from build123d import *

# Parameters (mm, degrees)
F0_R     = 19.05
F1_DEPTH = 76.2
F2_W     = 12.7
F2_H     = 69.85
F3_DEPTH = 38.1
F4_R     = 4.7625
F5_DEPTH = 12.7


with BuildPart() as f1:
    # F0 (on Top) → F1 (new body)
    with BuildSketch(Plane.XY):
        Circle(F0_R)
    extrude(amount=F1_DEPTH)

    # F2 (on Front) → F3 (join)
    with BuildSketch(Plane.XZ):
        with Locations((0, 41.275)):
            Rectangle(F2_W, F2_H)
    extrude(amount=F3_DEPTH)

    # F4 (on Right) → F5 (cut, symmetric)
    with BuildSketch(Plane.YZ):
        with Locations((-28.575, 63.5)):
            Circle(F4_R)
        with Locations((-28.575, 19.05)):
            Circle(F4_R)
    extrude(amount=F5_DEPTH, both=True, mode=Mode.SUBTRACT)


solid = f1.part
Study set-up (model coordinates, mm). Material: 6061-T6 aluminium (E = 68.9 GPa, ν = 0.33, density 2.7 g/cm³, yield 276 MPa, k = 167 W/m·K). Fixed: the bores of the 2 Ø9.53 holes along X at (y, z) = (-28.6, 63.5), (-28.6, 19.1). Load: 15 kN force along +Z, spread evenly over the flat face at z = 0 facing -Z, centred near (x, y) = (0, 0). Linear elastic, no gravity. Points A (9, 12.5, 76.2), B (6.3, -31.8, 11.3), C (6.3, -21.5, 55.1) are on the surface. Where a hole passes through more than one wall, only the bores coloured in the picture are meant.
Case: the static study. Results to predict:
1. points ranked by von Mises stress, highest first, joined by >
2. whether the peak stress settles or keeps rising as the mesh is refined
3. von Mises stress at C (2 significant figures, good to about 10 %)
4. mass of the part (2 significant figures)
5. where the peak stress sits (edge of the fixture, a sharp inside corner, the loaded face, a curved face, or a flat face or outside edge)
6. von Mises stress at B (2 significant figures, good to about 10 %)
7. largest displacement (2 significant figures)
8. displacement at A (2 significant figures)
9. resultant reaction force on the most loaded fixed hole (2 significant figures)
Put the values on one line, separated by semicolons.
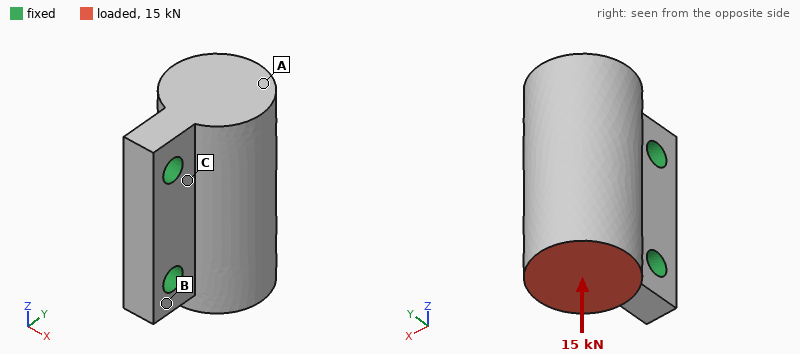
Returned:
C > B > A; keeps rising; 39 MPa; 280 g; edge of the fixture; 25 MPa; 36 µm; 23 µm; 11 kN
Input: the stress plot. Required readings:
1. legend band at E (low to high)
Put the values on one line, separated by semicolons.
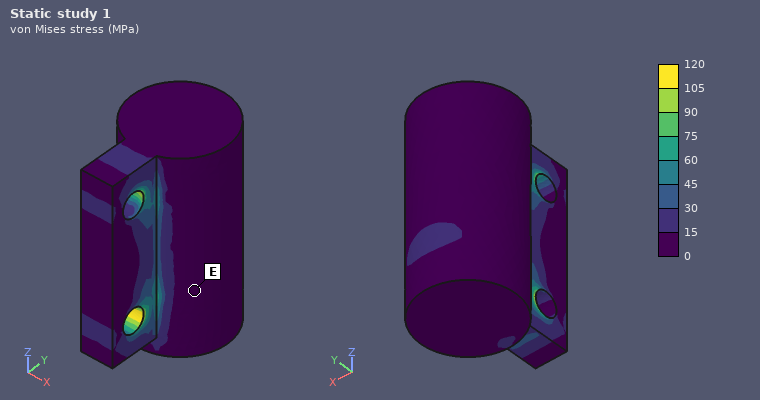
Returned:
0 to 15 MPa
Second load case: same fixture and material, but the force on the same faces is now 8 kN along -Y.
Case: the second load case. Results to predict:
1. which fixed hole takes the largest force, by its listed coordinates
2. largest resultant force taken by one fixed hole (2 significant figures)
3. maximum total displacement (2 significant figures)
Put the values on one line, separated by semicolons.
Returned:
(-28.6, 19.1); 11 kN; 29 µm
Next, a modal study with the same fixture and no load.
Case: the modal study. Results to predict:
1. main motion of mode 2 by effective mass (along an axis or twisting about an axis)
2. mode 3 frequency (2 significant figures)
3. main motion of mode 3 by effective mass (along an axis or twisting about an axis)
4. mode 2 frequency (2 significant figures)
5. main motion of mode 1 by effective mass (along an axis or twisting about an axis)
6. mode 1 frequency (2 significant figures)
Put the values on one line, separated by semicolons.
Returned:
twisting about Y; 8600 Hz; along Z; 7700 Hz; along X; 3000 Hz
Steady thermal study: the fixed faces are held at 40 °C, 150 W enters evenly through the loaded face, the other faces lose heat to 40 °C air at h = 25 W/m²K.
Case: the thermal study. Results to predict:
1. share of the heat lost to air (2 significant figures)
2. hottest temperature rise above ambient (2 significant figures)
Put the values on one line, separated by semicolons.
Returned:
3.1 %; 39 K
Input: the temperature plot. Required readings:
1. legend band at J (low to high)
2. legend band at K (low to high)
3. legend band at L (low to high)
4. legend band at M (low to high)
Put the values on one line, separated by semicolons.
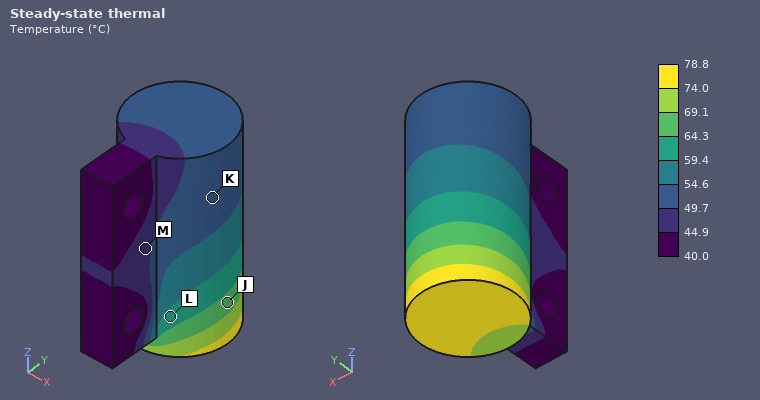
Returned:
64.3 to 69.1 °C; 49.7 to 54.6 °C; 59.4 to 64.3 °C; 44.9 to 49.7 °C
